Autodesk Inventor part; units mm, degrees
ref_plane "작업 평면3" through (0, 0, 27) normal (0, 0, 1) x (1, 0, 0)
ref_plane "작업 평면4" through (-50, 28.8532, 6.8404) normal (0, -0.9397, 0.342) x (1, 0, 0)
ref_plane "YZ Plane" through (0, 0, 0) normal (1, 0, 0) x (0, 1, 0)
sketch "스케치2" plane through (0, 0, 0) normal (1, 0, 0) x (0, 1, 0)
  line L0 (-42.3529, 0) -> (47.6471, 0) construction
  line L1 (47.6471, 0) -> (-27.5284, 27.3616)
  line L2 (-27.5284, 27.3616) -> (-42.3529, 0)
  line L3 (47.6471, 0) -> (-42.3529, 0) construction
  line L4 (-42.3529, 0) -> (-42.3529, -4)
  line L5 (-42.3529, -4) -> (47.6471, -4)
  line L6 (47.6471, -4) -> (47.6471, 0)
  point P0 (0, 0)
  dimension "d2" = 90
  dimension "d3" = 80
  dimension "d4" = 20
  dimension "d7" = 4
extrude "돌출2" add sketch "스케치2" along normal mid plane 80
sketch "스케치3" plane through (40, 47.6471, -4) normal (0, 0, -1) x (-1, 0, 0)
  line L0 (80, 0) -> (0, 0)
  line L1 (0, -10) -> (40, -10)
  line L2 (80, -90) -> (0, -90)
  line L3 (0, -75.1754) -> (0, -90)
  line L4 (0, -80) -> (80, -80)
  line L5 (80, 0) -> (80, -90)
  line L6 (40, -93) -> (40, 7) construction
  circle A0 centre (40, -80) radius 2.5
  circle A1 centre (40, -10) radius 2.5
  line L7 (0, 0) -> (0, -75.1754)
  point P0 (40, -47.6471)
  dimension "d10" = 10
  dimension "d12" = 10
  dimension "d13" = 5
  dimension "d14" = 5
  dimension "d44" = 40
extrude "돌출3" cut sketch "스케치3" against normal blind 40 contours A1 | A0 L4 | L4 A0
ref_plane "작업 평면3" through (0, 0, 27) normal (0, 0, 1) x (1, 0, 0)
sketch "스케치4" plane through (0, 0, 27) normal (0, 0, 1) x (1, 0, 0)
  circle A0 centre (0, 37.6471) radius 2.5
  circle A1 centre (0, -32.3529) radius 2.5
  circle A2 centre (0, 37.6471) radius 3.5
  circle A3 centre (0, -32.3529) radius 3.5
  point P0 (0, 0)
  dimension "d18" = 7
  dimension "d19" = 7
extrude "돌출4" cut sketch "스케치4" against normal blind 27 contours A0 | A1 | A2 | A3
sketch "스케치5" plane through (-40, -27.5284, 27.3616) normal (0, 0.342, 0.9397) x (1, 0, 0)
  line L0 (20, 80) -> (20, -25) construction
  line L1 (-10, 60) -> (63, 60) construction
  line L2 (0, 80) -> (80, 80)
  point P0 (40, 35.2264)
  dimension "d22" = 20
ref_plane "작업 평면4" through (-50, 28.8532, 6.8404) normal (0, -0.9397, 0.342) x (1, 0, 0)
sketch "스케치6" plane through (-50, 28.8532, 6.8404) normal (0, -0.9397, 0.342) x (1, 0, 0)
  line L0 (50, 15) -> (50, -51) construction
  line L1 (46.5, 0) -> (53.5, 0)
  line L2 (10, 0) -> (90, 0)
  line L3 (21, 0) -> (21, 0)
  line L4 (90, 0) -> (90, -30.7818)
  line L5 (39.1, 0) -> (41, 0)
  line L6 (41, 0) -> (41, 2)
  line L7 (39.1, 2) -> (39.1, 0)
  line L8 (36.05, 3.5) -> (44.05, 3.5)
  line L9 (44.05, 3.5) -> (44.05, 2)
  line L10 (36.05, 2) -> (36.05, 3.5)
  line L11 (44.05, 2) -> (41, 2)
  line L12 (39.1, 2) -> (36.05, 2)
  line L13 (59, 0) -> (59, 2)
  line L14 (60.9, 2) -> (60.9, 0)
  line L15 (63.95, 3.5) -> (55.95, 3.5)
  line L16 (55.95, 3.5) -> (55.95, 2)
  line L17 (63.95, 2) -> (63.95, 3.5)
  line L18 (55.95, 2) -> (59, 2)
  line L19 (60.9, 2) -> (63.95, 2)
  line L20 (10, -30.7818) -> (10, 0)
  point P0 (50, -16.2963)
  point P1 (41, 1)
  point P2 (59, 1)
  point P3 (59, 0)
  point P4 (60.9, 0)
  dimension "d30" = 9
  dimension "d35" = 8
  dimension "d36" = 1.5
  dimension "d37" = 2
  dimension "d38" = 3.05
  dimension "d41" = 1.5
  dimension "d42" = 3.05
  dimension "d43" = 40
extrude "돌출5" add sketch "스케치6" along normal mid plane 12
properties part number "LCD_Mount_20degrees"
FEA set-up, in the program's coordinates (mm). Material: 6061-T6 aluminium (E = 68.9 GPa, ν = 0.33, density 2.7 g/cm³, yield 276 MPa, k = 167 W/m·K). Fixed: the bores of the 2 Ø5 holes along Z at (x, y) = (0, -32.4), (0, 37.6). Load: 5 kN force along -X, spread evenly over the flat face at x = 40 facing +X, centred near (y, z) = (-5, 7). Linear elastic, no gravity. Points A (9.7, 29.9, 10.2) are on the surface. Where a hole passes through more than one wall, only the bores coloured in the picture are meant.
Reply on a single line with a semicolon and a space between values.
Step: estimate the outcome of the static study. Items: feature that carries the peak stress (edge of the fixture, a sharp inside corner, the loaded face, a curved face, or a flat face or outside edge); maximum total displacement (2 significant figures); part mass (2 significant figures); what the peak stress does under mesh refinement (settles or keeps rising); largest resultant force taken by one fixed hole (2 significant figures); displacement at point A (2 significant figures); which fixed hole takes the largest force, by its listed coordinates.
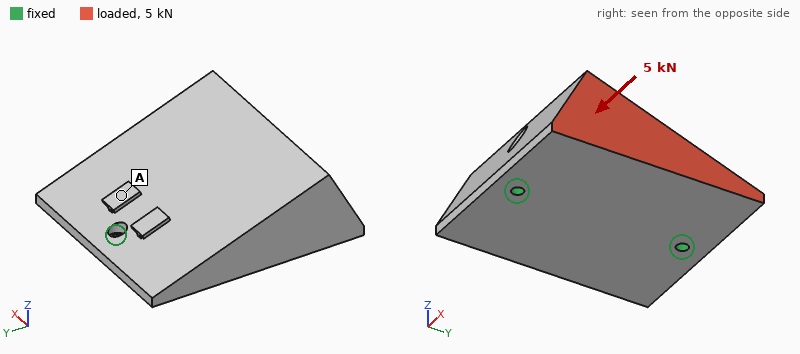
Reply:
edge of the fixture; 0.21 mm; 340 g; keeps rising; 3.0 kN; 0.062 mm; (0, -32.4)
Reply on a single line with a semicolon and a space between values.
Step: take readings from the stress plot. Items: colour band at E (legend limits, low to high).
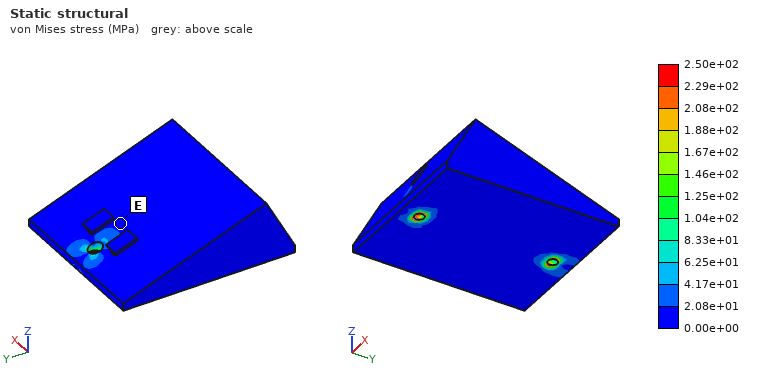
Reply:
0.00e+00 to 2.08e+01 MPa
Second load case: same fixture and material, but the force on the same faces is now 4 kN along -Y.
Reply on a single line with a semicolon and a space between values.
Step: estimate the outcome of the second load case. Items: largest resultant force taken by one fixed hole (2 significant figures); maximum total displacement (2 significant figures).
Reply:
3.1 kN; 17 µm
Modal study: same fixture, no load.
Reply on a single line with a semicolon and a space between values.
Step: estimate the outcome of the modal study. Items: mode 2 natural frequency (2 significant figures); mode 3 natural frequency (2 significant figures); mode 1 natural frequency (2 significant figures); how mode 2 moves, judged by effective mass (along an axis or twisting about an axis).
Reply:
4900 Hz; 7800 Hz; 1100 Hz; along Z
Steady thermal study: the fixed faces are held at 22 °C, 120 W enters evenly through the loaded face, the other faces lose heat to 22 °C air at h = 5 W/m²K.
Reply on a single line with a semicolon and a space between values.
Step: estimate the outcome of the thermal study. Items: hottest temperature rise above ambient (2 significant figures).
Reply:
37 K
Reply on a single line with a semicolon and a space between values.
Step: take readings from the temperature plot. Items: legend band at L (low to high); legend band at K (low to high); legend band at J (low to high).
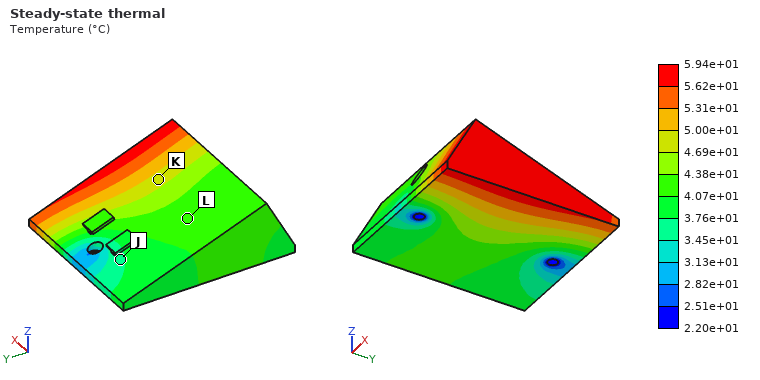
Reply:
4.07e+01 to 4.38e+01 °C; 4.69e+01 to 5.00e+01 °C; 3.45e+01 to 3.76e+01 °C
